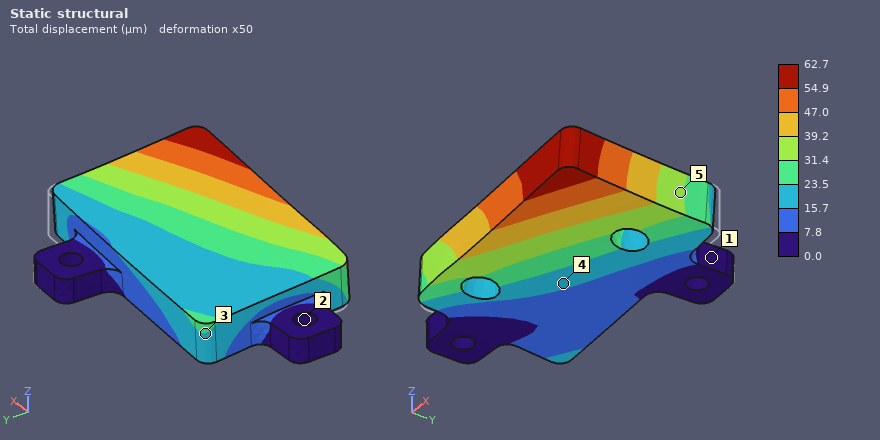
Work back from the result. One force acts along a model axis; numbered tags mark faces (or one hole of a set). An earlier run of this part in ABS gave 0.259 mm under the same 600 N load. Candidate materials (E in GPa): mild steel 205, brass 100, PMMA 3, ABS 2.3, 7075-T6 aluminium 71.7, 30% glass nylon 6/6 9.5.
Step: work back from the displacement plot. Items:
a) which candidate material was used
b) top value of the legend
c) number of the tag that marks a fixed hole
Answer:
30% glass nylon 6/6
62.7 µm
2
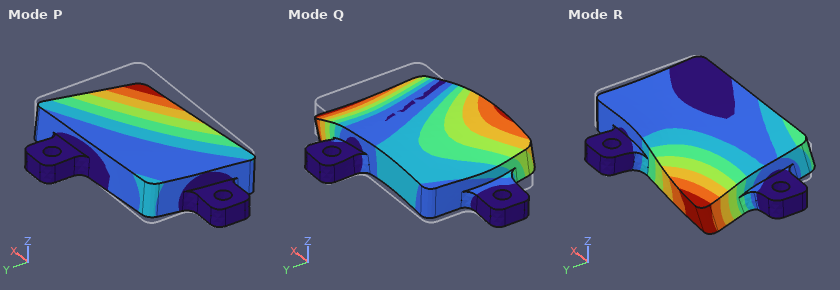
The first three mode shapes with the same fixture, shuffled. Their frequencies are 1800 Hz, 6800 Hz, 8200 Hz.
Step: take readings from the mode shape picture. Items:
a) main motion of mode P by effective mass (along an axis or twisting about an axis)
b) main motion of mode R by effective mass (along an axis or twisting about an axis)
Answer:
along Z
along Z
